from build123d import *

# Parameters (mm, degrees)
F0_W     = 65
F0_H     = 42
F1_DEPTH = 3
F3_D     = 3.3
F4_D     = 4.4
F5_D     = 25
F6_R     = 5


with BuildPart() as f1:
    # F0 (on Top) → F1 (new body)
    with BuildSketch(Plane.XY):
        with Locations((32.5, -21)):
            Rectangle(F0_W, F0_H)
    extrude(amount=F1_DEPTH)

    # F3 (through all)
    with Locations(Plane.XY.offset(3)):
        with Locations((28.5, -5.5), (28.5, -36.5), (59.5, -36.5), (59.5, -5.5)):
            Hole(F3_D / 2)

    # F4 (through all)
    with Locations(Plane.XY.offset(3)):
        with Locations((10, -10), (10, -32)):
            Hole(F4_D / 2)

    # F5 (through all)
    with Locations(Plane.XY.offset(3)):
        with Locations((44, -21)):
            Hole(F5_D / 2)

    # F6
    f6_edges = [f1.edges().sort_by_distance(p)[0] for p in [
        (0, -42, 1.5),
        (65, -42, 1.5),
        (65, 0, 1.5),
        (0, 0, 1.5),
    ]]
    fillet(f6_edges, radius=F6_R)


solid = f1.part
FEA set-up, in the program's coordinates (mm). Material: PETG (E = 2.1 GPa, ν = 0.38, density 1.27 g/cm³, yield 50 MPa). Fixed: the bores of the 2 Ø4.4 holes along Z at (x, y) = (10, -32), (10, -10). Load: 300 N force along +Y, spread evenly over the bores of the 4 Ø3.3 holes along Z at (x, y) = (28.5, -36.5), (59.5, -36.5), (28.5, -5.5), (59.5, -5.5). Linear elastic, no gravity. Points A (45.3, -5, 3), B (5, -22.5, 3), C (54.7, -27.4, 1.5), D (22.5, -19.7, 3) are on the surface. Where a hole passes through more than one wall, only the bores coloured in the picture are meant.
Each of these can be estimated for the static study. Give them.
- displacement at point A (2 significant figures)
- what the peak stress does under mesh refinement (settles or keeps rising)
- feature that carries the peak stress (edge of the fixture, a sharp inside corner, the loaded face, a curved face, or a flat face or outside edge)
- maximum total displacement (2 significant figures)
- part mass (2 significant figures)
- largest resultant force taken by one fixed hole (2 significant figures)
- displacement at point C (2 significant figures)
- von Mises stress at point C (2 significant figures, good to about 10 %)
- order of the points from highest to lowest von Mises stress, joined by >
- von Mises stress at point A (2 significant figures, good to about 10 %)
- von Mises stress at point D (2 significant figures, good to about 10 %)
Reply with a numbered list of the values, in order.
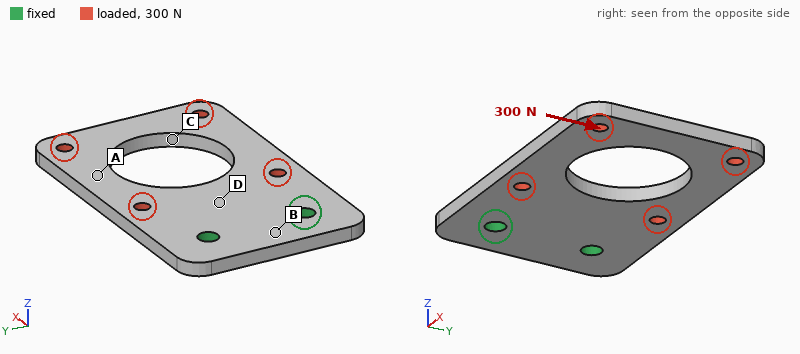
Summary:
1. 0.49 mm
2. keeps rising
3. edge of the fixture
4. 0.84 mm
5. 8.2 g
6. 430 N
7. 0.70 mm
8. 14 MPa
9. C > D > A > B
10. 7.6 MPa
11. 10 MPa
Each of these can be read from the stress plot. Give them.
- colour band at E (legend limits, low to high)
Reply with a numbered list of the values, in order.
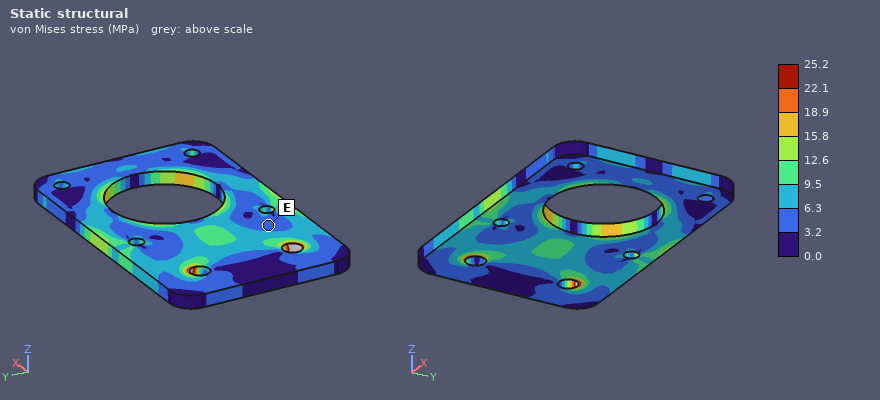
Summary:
1. 3.2 to 6.3 MPa
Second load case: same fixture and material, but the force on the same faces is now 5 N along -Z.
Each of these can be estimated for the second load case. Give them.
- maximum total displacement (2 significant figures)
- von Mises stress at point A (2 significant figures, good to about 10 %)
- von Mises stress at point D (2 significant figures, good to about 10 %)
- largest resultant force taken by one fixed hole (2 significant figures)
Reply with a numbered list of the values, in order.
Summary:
1. 0.83 mm
2. 1.4 MPa
3. 1.4 MPa
4. 2.5 N
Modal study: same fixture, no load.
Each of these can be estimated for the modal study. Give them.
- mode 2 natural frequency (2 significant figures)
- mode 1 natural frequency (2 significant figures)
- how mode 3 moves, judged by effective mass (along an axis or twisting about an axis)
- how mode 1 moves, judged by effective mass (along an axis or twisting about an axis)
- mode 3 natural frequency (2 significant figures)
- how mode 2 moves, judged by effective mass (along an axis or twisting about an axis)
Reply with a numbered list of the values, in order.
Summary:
1. 550 Hz
2. 220 Hz
3. along Z
4. along Z
5. 1200 Hz
6. twisting about X
